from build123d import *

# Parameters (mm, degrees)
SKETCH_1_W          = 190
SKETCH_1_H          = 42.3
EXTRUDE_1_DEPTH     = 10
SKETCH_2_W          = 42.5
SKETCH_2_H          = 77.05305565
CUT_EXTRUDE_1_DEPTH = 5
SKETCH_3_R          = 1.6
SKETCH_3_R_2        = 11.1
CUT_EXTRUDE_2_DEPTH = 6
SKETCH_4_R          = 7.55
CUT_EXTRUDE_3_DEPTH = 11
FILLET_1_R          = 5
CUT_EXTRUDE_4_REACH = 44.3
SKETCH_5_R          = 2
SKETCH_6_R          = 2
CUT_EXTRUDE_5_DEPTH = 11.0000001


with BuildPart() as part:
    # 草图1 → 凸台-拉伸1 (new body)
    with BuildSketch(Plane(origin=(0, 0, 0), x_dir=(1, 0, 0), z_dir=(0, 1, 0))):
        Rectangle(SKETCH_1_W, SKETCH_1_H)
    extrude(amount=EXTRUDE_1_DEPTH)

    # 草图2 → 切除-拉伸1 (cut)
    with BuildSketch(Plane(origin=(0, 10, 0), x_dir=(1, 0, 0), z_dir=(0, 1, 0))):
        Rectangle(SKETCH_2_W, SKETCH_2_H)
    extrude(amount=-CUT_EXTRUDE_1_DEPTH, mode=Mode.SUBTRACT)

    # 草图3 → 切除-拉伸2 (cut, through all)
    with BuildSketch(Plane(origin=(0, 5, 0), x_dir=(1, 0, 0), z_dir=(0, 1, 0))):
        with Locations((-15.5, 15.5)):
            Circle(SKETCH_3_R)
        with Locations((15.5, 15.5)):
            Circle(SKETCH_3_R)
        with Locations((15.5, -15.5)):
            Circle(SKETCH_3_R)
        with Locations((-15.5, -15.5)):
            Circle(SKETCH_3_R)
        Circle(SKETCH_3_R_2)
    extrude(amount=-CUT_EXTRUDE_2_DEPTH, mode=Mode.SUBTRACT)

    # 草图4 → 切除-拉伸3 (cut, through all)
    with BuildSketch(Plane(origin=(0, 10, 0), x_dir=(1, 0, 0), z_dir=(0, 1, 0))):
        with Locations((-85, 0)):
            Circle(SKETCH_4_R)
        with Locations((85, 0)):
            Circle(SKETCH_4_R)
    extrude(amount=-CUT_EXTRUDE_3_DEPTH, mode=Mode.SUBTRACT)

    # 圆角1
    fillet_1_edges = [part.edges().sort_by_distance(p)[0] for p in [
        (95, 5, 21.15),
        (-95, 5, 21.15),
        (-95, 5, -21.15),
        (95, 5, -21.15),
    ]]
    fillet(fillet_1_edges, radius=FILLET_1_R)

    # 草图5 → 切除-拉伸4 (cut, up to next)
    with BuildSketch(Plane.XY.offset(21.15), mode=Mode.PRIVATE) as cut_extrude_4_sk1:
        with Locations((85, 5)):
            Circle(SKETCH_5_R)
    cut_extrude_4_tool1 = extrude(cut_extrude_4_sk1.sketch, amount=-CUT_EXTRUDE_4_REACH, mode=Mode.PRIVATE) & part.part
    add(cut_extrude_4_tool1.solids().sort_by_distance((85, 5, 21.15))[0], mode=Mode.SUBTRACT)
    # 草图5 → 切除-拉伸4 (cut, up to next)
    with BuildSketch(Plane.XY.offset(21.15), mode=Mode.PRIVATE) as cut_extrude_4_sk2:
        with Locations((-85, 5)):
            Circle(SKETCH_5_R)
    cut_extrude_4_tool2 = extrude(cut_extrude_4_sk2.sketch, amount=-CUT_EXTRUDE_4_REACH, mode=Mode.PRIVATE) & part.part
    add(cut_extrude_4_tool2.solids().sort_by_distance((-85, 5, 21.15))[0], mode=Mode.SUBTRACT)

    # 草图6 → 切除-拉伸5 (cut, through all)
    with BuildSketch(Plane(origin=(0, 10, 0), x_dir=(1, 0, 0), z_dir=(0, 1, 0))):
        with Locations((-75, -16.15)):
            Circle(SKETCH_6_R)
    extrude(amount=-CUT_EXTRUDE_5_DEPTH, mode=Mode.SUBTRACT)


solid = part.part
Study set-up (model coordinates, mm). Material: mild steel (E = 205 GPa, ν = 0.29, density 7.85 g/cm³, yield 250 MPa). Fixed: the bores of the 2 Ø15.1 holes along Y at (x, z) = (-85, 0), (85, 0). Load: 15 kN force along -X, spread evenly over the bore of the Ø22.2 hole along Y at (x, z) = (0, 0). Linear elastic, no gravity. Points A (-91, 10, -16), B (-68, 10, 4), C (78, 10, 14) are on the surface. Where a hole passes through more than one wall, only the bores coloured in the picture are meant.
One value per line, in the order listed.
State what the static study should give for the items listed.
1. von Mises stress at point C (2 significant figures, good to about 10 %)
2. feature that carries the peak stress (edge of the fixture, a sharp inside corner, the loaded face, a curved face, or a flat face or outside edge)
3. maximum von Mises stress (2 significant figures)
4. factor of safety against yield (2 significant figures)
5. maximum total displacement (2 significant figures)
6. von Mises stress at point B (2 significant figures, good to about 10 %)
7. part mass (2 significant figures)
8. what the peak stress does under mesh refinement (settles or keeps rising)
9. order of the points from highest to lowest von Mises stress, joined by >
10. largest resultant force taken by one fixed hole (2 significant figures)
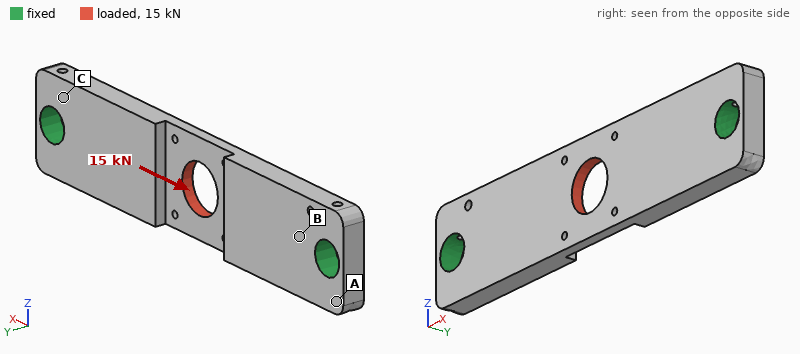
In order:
13 MPa
a curved face
150 MPa
1.7
13 µm
24 MPa
510 g
settles
B > C > A
7.5 kN
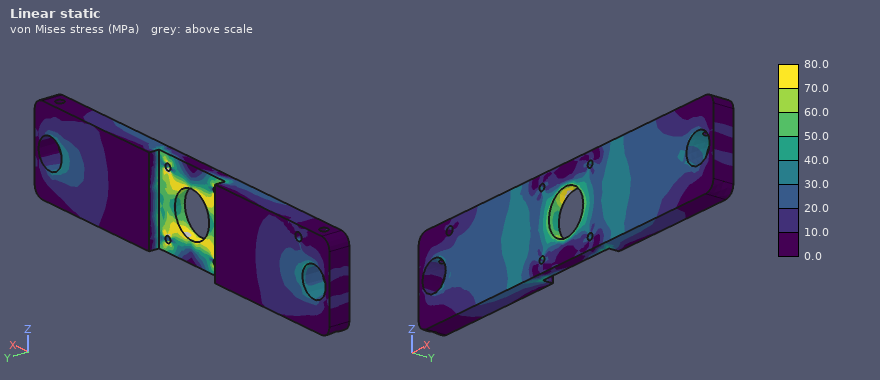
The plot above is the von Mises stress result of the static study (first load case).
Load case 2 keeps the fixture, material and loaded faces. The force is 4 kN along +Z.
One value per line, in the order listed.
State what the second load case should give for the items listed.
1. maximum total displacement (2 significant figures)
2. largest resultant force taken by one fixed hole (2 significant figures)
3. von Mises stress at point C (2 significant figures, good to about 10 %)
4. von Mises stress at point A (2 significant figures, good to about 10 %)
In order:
27 µm
2.0 kN
21 MPa
12 MPa
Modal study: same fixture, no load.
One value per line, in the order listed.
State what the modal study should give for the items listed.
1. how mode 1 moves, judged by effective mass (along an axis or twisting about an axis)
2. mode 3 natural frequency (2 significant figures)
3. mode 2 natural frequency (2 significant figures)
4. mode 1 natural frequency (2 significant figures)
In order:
along Y
4800 Hz
3800 Hz
2000 Hz
